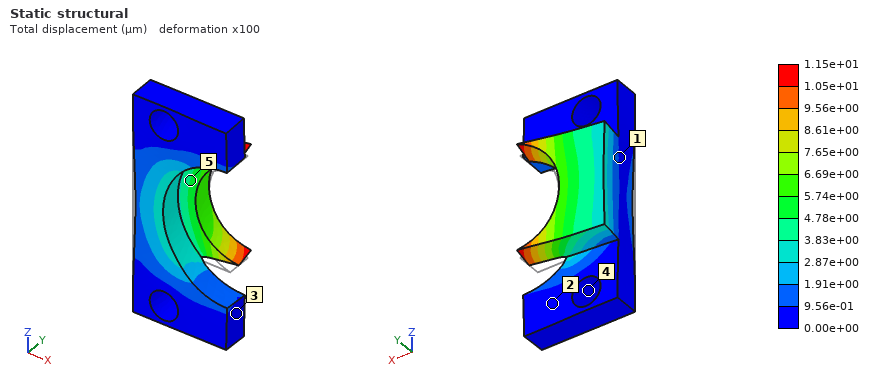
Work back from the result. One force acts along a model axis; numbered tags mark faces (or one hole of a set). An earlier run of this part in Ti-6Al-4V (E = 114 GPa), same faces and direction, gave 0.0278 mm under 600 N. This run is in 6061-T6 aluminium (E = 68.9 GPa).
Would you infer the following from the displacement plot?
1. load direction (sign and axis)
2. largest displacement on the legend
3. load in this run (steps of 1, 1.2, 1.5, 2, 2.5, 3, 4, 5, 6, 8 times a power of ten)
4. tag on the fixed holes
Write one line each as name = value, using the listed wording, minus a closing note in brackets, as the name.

load direction = +Y
largest displacement on the legend = 1.15e+01 µm
load in this run = 150 N
tag on the fixed holes = 4
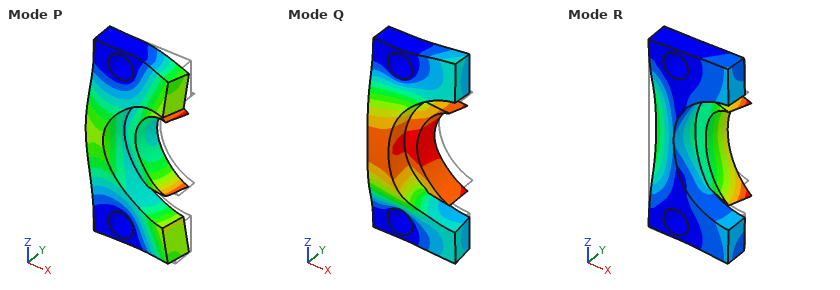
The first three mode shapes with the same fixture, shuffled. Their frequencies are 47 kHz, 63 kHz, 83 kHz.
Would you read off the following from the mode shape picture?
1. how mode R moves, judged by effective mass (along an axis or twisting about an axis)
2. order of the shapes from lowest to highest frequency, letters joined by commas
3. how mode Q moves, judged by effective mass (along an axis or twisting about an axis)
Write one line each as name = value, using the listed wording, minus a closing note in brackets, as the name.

how mode R moves, judged by effective mass = along X
order of the shapes from lowest to highest frequency, letters joined by commas = R, Q, P
how mode Q moves, judged by effective mass = along Y
